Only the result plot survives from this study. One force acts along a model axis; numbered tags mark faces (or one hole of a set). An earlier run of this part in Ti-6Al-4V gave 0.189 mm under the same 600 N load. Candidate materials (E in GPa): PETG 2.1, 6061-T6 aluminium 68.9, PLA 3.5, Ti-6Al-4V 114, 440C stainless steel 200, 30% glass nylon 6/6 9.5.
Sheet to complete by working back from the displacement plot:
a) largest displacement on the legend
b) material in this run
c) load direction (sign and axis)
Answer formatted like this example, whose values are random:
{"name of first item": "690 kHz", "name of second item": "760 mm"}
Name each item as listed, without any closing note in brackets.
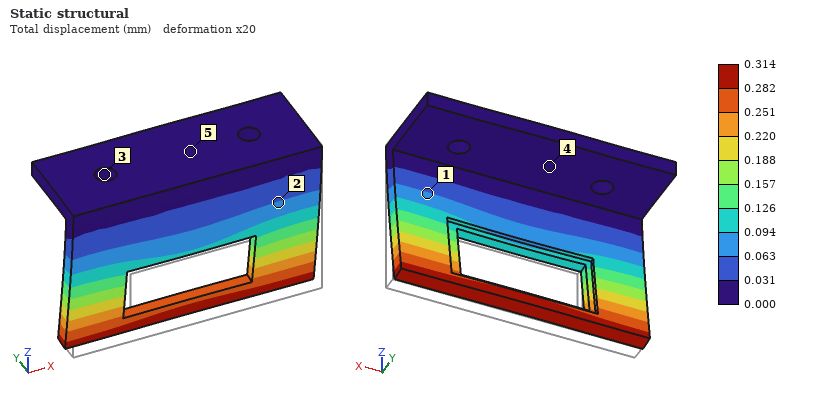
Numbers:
{"largest displacement on the legend": "0.314 mm", "material in this run": "6061-T6 aluminium", "load direction": "+Y"}
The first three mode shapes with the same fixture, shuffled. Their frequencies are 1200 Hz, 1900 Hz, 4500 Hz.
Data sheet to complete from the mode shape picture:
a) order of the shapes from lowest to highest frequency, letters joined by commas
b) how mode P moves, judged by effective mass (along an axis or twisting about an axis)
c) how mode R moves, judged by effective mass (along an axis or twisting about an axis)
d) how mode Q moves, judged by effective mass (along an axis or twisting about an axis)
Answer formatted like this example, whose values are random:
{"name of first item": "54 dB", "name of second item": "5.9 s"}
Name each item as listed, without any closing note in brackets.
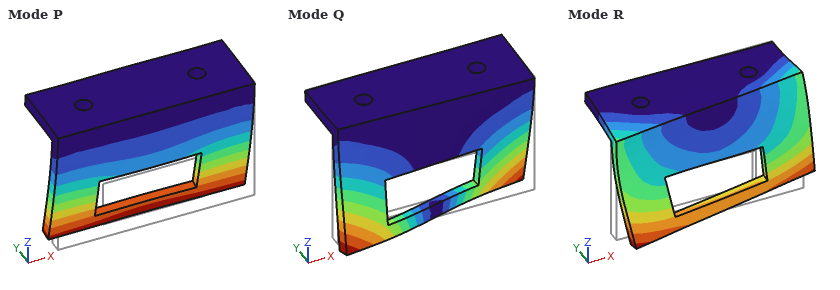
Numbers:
{"order of the shapes from lowest to highest frequency, letters joined by commas": "P, Q, R", "how mode P moves, judged by effective mass": "along Y", "how mode R moves, judged by effective mass": "along X", "how mode Q moves, judged by effective mass": "twisting about Z"}
